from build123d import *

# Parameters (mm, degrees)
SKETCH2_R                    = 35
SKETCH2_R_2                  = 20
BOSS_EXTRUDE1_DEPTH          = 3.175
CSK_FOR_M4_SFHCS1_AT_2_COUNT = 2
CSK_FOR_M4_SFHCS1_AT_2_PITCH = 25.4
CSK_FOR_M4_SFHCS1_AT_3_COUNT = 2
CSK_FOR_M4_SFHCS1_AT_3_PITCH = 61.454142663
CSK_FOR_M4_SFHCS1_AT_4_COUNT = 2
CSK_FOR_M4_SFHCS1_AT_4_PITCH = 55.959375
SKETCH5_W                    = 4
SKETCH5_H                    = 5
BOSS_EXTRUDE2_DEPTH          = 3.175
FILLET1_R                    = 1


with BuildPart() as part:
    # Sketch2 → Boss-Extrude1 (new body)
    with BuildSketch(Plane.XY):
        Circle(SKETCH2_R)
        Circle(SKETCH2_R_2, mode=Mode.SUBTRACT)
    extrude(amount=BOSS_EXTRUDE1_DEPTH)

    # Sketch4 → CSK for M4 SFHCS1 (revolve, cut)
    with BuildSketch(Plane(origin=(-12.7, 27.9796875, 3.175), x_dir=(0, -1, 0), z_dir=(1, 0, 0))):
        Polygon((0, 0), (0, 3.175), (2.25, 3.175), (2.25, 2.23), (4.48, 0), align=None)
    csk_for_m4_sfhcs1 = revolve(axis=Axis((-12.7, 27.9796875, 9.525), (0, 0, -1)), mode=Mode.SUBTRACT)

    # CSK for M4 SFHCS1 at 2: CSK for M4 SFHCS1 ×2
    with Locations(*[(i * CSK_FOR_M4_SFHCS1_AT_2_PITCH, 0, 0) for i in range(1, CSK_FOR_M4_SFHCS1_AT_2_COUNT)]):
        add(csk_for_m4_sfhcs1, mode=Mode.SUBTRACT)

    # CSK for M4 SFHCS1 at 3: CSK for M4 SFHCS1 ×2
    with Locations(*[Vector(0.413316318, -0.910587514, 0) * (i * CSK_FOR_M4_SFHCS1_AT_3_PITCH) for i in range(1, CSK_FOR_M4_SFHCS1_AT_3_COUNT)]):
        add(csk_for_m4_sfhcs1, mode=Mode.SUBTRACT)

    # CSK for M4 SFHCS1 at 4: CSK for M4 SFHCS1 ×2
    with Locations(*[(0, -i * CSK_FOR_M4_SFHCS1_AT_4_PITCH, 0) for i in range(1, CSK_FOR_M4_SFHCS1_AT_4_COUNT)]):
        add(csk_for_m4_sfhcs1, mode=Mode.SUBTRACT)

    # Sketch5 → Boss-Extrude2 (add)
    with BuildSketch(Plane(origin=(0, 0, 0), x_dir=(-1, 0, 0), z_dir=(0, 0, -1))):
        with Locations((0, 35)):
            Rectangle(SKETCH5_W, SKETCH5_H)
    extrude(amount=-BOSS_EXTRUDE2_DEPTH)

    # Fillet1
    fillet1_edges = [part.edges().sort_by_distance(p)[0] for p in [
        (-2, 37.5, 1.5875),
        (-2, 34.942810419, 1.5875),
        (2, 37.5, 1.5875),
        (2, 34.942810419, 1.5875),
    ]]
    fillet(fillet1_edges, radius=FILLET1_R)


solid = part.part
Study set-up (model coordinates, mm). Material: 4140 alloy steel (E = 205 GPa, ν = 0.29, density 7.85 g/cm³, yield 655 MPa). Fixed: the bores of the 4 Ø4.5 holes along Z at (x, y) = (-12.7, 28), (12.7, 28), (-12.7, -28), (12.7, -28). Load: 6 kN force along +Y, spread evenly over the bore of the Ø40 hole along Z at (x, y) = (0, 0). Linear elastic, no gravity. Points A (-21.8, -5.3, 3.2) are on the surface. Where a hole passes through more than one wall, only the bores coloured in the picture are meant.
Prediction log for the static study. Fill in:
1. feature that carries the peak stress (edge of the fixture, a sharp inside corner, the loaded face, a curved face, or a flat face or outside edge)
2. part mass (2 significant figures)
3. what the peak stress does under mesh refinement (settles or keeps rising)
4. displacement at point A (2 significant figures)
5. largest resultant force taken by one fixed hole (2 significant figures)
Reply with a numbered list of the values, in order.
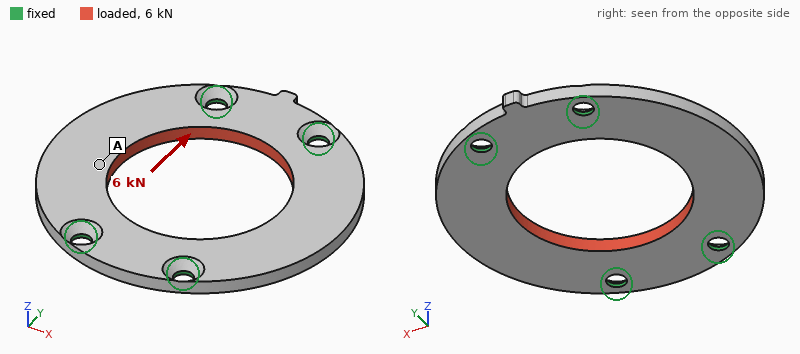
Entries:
1. edge of the fixture
2. 62 g
3. keeps rising
4. 5.2 µm
5. 1.5 kN
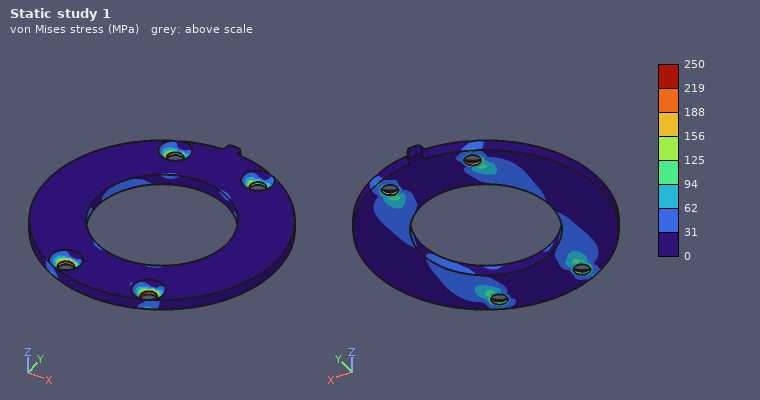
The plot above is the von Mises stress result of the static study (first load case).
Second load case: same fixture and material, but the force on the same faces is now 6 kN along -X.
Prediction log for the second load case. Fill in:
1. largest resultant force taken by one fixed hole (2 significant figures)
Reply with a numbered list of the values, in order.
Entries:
1. 1.5 kN
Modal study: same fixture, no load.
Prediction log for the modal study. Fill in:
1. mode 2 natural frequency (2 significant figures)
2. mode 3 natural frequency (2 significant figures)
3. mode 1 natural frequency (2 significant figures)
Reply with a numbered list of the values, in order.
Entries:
1. 2800 Hz
2. 8000 Hz
3. 2800 Hz
